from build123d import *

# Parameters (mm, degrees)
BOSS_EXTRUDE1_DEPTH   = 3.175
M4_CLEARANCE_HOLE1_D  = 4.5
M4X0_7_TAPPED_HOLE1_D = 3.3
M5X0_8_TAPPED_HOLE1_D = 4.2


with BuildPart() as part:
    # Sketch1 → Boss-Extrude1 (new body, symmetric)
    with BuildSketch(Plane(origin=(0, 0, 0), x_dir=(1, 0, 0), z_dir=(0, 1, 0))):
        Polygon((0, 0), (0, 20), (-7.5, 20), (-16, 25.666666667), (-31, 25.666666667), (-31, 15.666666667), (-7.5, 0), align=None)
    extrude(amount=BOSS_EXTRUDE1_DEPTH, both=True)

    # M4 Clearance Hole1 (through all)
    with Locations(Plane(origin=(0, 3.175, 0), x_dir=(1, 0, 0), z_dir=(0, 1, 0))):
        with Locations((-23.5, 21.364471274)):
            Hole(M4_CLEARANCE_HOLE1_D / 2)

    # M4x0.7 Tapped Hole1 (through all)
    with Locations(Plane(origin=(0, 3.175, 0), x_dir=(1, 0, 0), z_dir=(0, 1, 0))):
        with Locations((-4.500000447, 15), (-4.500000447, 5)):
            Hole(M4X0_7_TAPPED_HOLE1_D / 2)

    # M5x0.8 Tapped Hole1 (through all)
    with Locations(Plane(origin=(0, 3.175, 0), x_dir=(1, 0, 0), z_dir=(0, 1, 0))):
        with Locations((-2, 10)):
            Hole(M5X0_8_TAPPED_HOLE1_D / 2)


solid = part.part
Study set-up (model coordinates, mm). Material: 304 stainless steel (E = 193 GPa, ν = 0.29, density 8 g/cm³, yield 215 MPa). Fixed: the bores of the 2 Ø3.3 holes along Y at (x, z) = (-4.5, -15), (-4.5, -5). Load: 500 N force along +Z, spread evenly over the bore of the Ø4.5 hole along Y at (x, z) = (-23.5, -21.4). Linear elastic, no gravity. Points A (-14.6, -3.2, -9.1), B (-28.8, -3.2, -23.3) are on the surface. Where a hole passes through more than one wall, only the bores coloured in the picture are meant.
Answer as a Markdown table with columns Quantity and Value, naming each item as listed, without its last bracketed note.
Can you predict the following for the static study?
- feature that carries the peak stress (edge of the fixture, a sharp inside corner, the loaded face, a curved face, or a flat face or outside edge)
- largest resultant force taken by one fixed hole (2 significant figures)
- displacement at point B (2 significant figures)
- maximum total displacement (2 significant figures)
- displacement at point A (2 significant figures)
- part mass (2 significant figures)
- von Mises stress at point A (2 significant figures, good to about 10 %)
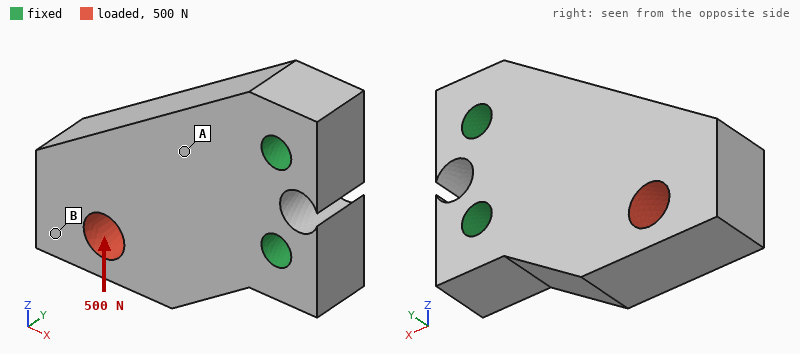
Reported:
| Quantity | Value |
|---|---|
| feature that carries the peak stress | edge of the fixture |
| largest resultant force taken by one fixed hole | 820 N |
| displacement at point B | 5.5 µm |
| maximum total displacement | 6.0 µm |
| displacement at point A | 1.3 µm |
| part mass | 25 g |
| von Mises stress at point A | 14 MPa |
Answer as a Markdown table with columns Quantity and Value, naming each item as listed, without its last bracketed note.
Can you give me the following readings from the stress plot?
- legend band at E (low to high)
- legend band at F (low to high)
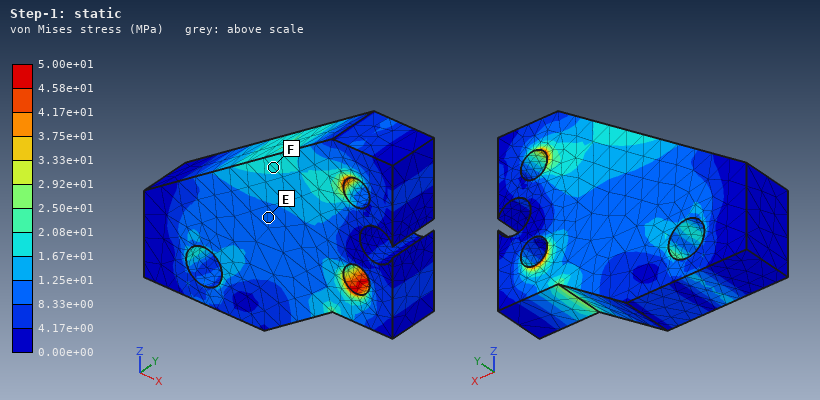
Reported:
| Quantity | Value |
|---|---|
| legend band at E | 8.33e+00 to 1.25e+01 MPa |
| legend band at F | 1.67e+01 to 2.08e+01 MPa |
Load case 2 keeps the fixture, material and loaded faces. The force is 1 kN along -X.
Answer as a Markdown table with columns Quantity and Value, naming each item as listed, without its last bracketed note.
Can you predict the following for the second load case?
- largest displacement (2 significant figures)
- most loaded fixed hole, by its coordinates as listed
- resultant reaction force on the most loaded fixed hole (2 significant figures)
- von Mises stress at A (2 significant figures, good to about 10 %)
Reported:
| Quantity | Value |
|---|---|
| largest displacement | 7.7 µm |
| most loaded fixed hole, by its coordinates as listed | (-4.5, -15) |
| resultant reaction force on the most loaded fixed hole | 1.4 kN |
| von Mises stress at A | 8.5 MPa |
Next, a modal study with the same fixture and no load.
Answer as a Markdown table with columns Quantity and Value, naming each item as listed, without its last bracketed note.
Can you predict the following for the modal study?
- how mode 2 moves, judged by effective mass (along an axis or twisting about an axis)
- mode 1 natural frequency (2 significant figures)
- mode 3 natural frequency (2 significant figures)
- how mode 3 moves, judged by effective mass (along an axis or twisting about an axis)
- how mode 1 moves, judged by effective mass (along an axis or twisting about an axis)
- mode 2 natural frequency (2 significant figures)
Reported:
| Quantity | Value |
|---|---|
| how mode 2 moves, judged by effective mass | along Z |
| mode 1 natural frequency | 7700 Hz |
| mode 3 natural frequency | 23 kHz |
| how mode 3 moves, judged by effective mass | twisting about X |
| how mode 1 moves, judged by effective mass | along Y |
| mode 2 natural frequency | 16 kHz |
